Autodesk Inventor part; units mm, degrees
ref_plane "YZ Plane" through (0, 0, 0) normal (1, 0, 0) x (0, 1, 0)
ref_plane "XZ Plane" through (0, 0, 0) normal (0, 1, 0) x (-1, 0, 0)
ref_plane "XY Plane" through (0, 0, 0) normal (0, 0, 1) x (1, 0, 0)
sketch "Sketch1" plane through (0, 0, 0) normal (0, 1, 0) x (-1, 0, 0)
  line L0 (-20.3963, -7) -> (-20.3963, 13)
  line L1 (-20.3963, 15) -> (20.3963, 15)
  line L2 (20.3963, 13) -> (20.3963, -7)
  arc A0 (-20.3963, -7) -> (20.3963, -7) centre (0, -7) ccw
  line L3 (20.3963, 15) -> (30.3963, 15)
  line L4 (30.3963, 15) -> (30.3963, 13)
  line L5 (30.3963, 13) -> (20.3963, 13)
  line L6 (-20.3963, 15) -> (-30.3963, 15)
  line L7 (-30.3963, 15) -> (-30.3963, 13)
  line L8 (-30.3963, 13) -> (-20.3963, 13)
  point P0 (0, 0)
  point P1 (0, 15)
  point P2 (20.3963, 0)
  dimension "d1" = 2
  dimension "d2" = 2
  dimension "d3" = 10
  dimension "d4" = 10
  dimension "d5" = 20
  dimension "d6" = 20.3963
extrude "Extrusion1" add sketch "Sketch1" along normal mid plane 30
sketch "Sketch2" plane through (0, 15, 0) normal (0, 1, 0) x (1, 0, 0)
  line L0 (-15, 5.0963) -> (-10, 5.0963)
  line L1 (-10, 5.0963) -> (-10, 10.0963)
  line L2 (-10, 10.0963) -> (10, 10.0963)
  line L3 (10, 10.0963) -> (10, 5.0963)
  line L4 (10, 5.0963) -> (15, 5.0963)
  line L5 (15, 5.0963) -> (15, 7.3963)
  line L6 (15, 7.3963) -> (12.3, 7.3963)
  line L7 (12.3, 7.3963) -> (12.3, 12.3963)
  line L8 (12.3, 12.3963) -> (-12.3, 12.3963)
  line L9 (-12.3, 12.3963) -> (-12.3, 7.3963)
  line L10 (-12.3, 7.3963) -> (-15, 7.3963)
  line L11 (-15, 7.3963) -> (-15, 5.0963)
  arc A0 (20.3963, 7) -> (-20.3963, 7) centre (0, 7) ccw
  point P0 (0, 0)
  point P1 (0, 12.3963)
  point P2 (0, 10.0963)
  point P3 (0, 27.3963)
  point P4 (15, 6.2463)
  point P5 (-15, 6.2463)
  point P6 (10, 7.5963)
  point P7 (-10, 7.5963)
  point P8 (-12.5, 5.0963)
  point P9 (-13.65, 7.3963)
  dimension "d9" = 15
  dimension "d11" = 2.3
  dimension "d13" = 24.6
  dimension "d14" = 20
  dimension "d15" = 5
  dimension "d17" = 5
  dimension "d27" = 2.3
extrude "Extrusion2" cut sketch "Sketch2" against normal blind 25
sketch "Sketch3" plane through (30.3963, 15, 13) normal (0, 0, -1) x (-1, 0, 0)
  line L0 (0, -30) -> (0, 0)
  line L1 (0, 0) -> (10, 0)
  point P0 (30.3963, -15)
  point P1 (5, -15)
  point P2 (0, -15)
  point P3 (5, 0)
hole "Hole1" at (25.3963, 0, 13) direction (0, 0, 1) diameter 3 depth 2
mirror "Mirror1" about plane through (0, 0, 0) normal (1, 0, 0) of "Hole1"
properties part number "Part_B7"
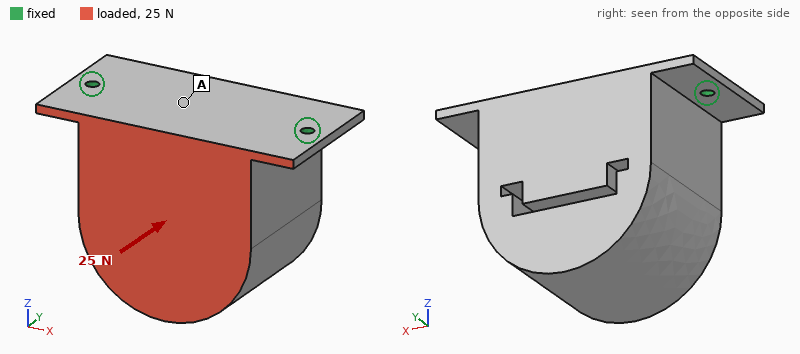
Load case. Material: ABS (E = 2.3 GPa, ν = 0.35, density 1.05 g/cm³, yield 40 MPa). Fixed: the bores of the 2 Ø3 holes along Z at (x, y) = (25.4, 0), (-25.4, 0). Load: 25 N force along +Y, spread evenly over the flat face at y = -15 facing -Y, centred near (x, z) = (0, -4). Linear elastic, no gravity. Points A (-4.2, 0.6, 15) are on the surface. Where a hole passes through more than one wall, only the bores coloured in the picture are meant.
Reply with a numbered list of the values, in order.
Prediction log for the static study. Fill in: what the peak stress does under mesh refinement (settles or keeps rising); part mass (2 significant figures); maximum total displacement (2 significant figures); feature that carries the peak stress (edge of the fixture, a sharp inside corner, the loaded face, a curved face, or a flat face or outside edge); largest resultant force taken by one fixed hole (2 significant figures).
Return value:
1. keeps rising
2. 48 g
3. 0.81 mm
4. edge of the fixture
5. 13 N
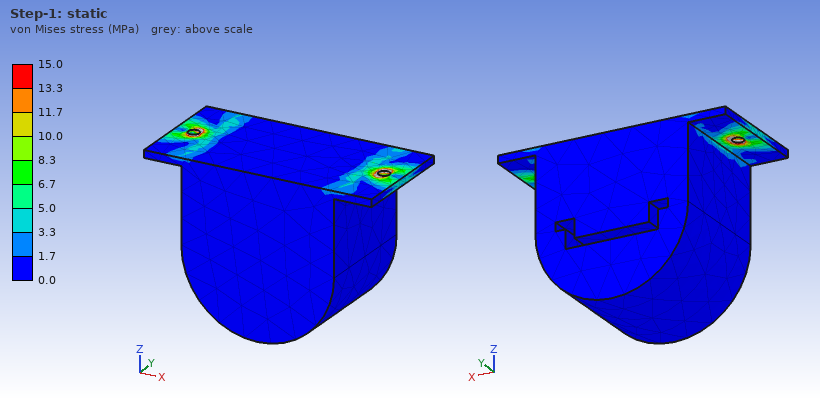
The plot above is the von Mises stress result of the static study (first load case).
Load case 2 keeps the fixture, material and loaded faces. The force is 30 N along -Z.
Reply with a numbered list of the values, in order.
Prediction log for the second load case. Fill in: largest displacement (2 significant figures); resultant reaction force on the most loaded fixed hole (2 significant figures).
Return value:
1. 0.82 mm
2. 17 N
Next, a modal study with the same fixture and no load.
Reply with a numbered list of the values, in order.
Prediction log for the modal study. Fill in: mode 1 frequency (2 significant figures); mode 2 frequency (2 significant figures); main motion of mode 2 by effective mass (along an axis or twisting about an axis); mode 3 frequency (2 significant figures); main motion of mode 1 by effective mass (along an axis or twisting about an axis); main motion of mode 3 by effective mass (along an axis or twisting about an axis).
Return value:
1. 160 Hz
2. 930 Hz
3. along X
4. 1000 Hz
5. along Y
6. along Z
